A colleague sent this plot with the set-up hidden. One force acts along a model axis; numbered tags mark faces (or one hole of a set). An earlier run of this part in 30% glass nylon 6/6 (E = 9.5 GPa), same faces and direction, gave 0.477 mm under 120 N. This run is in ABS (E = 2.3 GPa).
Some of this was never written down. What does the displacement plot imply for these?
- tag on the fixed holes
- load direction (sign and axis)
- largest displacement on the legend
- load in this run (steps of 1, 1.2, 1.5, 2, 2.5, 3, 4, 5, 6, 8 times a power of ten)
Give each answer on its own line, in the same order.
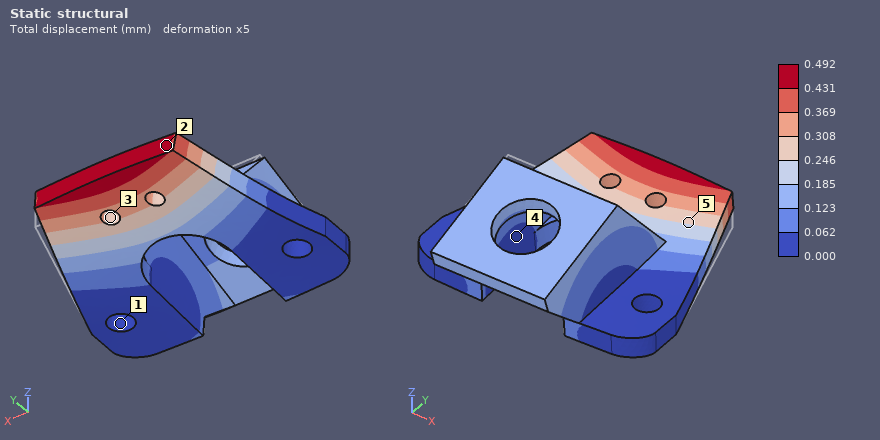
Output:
1
+Z
0.492 mm
30 N
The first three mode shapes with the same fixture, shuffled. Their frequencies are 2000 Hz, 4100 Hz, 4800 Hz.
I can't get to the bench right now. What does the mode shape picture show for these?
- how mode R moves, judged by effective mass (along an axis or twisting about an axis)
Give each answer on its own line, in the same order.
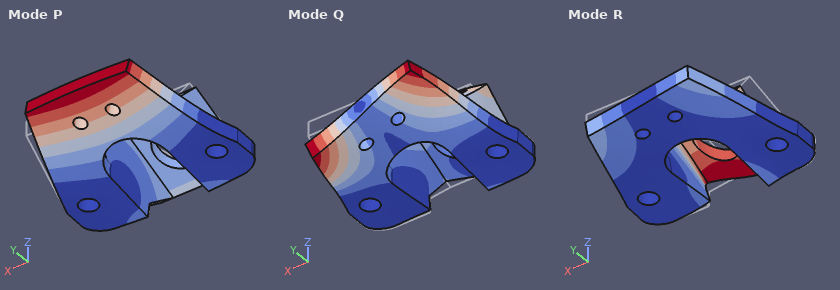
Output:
along X
